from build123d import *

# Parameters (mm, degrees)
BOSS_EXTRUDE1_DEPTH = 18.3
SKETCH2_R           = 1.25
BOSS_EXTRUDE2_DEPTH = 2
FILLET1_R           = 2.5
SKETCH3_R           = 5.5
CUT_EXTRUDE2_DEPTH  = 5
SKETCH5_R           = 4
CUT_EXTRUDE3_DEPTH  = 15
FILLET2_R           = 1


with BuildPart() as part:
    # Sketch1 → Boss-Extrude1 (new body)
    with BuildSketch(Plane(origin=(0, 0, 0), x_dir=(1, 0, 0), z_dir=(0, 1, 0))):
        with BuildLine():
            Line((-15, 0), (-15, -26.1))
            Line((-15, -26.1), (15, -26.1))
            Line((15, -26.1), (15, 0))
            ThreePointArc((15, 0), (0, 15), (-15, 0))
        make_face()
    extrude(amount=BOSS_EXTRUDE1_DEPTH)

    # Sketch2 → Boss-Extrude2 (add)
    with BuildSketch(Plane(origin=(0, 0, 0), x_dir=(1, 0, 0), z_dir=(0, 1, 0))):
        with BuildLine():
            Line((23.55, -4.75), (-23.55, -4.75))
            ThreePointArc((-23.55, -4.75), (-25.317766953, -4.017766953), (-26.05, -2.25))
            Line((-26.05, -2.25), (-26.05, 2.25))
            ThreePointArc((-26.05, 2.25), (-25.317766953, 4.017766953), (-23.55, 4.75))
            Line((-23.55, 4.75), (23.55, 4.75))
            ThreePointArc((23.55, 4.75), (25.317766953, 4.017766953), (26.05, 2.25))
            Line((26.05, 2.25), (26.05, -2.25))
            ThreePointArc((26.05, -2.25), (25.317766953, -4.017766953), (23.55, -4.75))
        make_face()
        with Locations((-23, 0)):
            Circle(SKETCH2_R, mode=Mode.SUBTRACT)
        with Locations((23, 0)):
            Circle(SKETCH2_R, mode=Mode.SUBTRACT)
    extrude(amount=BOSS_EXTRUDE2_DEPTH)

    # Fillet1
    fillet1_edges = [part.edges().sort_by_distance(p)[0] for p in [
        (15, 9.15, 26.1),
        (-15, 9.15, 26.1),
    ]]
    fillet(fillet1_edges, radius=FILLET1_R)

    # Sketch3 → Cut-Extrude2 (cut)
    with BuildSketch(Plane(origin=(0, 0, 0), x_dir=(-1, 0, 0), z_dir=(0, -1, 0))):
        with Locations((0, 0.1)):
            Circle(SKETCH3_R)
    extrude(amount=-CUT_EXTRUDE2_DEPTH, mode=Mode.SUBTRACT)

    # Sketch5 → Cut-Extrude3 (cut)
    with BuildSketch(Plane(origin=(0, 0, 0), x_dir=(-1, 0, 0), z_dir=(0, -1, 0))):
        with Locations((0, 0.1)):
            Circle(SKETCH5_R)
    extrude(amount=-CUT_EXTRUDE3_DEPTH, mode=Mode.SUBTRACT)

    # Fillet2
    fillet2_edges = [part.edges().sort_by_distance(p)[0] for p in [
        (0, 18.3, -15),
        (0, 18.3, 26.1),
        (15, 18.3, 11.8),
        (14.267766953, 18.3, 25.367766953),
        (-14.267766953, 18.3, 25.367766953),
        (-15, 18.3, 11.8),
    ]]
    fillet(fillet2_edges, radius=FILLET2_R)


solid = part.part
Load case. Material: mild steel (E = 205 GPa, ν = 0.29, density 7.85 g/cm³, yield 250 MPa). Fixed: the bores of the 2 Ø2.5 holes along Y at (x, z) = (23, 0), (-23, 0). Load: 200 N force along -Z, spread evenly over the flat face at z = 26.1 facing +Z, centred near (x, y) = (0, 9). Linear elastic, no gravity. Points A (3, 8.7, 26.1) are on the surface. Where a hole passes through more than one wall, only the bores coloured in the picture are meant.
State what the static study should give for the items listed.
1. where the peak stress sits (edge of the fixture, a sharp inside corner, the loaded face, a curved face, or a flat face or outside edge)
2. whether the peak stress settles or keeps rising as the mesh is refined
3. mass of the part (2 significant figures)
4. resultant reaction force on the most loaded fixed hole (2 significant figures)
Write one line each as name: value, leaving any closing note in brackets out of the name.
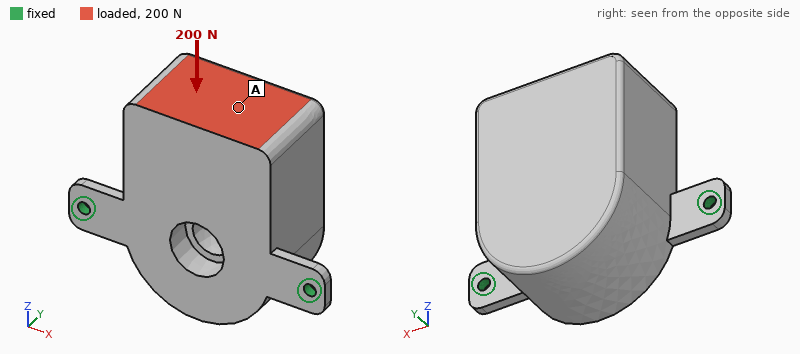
where the peak stress sits: edge of the fixture
whether the peak stress settles or keeps rising as the mesh is refined: keeps rising
mass of the part: 160 g
resultant reaction force on the most loaded fixed hole: 100 N
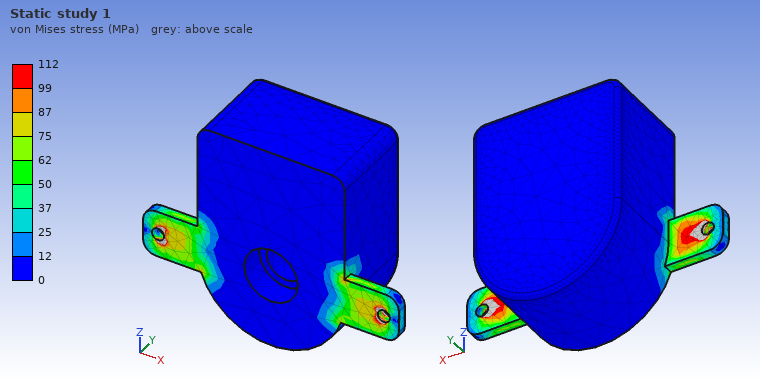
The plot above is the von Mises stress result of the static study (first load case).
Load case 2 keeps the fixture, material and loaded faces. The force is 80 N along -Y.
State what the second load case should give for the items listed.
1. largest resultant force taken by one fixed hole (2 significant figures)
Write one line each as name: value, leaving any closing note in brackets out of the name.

largest resultant force taken by one fixed hole: 44 N
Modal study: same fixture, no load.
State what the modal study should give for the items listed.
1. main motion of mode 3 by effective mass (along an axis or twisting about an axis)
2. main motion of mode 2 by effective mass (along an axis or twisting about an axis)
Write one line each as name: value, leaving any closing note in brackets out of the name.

main motion of mode 3 by effective mass: along X
main motion of mode 2 by effective mass: along Y
